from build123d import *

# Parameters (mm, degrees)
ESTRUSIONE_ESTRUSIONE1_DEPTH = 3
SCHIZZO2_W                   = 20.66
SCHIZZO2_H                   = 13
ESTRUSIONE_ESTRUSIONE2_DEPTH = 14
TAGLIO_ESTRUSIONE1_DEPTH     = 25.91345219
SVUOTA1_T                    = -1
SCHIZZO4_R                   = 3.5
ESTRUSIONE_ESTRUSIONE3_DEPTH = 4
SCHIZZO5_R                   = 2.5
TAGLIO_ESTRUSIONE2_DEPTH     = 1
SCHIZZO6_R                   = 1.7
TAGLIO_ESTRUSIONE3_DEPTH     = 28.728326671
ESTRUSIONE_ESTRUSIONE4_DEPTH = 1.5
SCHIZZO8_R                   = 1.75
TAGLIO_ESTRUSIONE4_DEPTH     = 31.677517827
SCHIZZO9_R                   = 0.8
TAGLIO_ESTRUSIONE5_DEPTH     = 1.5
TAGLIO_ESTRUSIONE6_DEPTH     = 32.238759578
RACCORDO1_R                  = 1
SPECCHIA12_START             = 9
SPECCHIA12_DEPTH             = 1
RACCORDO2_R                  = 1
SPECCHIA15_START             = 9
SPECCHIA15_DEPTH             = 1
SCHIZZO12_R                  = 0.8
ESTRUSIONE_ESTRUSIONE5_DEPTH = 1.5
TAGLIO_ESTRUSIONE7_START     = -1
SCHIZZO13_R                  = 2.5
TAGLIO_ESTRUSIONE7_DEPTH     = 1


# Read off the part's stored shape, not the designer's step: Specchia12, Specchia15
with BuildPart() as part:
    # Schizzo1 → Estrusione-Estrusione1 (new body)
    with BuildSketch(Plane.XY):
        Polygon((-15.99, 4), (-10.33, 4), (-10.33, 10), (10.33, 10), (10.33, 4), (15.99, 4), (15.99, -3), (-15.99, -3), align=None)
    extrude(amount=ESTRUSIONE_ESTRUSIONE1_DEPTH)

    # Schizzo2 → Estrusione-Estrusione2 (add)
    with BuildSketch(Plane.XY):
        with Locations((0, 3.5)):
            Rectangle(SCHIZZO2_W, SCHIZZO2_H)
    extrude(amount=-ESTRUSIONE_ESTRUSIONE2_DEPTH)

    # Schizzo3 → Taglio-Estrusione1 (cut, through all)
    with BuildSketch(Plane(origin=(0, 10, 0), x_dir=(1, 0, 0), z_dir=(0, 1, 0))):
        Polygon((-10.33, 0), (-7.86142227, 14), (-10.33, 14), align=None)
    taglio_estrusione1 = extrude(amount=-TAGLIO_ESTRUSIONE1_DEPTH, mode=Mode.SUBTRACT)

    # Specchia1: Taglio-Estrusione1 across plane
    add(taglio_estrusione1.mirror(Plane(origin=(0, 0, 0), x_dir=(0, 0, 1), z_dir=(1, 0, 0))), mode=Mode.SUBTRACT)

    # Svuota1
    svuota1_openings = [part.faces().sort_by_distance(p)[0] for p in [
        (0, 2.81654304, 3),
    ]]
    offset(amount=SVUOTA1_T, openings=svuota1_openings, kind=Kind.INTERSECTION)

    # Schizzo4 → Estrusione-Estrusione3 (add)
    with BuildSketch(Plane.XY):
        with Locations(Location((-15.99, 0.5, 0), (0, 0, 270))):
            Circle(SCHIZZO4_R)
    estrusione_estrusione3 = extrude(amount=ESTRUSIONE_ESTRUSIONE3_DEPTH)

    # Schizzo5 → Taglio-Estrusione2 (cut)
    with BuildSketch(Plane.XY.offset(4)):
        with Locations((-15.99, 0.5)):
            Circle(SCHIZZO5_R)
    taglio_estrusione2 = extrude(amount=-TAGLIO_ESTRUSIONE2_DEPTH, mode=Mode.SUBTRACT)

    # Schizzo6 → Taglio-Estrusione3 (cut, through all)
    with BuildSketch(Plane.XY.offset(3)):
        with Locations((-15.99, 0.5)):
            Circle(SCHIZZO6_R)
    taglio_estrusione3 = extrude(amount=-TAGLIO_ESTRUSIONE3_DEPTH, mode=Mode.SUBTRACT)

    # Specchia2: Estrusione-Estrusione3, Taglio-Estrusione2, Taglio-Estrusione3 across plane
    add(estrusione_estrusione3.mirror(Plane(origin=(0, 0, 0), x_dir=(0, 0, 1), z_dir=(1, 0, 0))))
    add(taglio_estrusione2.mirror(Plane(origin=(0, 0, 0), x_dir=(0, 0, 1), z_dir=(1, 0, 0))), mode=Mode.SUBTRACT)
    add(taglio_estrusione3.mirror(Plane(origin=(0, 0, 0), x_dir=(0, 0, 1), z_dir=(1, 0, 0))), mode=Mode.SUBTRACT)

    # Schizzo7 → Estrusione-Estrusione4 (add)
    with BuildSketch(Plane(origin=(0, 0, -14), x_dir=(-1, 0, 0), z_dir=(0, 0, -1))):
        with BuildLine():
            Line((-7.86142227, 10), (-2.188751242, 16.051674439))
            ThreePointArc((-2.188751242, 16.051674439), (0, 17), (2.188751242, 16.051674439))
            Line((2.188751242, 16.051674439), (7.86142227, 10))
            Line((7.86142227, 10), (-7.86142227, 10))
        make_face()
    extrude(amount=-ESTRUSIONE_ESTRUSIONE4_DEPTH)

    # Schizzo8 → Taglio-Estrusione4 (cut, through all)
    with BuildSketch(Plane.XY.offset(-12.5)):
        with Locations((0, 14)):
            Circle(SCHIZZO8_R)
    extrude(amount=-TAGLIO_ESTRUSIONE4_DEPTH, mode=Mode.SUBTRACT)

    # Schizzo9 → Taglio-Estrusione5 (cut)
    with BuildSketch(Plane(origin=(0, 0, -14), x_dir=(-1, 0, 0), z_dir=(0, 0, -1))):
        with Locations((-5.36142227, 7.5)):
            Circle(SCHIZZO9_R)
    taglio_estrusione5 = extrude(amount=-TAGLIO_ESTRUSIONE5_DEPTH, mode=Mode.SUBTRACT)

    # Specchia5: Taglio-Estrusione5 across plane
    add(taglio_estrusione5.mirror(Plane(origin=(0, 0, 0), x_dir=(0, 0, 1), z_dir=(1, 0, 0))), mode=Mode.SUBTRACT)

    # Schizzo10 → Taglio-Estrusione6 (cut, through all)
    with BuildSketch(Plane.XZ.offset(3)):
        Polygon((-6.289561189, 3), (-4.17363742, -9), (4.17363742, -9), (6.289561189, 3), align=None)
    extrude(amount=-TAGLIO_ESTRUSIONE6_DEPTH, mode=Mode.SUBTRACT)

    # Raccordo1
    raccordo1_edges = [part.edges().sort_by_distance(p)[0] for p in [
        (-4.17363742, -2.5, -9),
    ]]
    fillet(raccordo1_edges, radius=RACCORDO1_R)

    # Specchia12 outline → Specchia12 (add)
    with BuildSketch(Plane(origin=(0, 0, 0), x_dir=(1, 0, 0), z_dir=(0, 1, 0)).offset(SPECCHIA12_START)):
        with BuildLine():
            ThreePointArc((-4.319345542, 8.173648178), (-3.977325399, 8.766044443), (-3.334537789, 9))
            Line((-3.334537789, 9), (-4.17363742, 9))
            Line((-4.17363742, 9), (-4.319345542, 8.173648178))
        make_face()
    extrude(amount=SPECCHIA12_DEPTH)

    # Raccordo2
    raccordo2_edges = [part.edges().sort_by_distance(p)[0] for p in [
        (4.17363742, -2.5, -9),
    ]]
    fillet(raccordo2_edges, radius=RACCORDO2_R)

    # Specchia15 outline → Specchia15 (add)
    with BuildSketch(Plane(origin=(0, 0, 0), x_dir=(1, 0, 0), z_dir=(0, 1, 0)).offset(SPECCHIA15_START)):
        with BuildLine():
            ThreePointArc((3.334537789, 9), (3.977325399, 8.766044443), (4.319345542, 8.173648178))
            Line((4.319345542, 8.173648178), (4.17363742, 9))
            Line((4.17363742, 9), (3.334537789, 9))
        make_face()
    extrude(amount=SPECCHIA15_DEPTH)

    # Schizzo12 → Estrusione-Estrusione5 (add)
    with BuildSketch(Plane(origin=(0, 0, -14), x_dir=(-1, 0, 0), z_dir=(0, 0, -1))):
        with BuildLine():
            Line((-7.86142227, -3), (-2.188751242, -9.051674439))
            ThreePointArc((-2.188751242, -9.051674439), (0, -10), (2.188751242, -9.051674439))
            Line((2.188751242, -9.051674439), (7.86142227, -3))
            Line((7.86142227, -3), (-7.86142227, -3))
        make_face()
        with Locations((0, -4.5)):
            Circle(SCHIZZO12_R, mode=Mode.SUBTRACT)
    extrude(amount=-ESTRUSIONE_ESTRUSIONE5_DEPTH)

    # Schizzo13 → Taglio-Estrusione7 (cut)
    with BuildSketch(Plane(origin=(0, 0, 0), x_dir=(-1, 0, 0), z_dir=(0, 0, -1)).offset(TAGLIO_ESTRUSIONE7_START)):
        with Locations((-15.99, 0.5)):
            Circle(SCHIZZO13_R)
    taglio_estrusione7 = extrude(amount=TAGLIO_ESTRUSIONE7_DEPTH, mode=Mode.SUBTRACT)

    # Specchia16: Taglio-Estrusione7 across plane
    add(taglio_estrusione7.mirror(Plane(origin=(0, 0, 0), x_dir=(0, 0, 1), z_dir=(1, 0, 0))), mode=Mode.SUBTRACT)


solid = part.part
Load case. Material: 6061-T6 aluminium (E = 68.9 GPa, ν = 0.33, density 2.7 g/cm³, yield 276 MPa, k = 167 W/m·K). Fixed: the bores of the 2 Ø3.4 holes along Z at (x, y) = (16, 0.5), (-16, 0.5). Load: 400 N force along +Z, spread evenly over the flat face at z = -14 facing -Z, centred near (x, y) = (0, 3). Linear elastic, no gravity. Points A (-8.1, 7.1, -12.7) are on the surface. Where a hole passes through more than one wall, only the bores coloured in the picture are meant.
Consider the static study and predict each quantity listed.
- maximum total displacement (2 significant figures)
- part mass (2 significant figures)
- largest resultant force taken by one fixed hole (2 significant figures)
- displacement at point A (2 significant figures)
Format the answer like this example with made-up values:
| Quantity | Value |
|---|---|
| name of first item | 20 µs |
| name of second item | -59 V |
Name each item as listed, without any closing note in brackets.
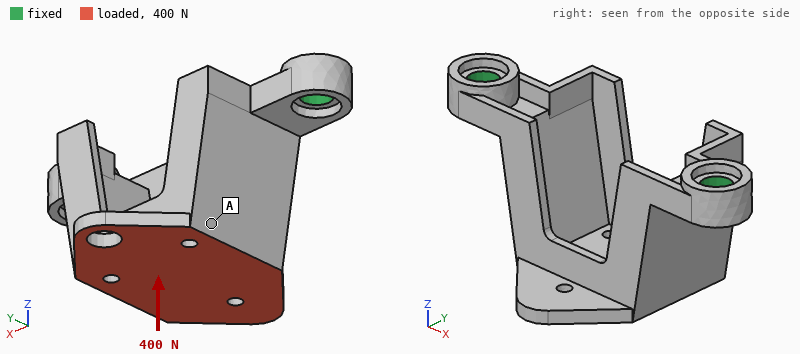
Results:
| Quantity | Value |
|---|---|
| maximum total displacement | 0.17 mm |
| part mass | 3.6 g |
| largest resultant force taken by one fixed hole | 220 N |
| displacement at point A | 0.10 mm |
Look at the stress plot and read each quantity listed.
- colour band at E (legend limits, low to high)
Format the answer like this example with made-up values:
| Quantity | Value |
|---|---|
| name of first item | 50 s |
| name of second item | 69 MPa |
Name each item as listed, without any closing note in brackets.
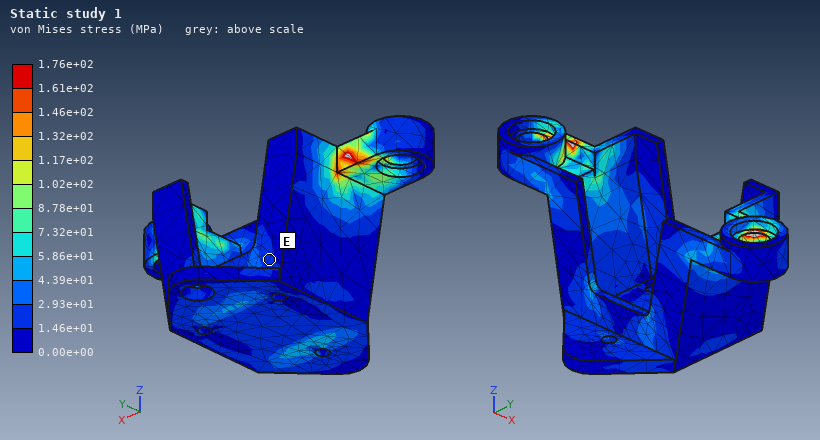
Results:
| Quantity | Value |
|---|---|
| colour band at E | 1.46e+01 to 2.93e+01 MPa |
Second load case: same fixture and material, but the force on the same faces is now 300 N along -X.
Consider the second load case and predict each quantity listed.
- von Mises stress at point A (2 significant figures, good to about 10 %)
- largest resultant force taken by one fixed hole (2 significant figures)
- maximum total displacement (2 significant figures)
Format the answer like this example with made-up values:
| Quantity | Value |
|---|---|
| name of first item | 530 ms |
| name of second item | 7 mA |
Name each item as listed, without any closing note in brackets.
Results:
| Quantity | Value |
|---|---|
| von Mises stress at point A | 18 MPa |
| largest resultant force taken by one fixed hole | 240 N |
| maximum total displacement | 72 µm |
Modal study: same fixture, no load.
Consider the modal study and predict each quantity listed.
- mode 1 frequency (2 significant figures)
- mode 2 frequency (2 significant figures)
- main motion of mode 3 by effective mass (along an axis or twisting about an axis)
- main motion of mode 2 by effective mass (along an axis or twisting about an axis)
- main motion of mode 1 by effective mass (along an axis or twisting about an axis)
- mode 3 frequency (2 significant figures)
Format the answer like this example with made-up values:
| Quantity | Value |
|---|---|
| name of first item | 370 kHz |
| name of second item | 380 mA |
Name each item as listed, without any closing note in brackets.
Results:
| Quantity | Value |
|---|---|
| mode 1 frequency | 3300 Hz |
| mode 2 frequency | 6500 Hz |
| main motion of mode 3 by effective mass | along X |
| main motion of mode 2 by effective mass | along X |
| main motion of mode 1 by effective mass | along Y |
| mode 3 frequency | 11 kHz |
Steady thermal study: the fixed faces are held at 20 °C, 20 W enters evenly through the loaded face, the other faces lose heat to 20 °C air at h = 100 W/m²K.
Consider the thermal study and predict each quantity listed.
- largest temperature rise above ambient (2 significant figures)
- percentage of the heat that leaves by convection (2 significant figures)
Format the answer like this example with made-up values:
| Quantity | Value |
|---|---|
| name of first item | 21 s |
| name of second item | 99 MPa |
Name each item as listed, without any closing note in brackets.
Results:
| Quantity | Value |
|---|---|
| largest temperature rise above ambient | 58 K |
| percentage of the heat that leaves by convection | 38 % |
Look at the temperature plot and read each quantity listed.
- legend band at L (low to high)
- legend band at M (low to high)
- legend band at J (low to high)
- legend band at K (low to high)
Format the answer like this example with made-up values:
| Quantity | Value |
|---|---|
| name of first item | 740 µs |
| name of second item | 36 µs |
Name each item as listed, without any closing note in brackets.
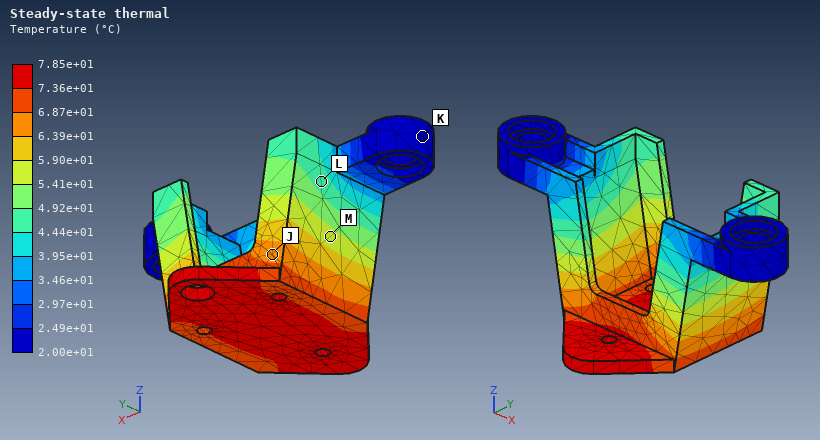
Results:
| Quantity | Value |
|---|---|
| legend band at L | 4.44e+01 to 4.92e+01 °C |
| legend band at M | 5.41e+01 to 5.90e+01 °C |
| legend band at J | 6.39e+01 to 6.87e+01 °C |
| legend band at K | 2.00e+01 to 2.49e+01 °C |
